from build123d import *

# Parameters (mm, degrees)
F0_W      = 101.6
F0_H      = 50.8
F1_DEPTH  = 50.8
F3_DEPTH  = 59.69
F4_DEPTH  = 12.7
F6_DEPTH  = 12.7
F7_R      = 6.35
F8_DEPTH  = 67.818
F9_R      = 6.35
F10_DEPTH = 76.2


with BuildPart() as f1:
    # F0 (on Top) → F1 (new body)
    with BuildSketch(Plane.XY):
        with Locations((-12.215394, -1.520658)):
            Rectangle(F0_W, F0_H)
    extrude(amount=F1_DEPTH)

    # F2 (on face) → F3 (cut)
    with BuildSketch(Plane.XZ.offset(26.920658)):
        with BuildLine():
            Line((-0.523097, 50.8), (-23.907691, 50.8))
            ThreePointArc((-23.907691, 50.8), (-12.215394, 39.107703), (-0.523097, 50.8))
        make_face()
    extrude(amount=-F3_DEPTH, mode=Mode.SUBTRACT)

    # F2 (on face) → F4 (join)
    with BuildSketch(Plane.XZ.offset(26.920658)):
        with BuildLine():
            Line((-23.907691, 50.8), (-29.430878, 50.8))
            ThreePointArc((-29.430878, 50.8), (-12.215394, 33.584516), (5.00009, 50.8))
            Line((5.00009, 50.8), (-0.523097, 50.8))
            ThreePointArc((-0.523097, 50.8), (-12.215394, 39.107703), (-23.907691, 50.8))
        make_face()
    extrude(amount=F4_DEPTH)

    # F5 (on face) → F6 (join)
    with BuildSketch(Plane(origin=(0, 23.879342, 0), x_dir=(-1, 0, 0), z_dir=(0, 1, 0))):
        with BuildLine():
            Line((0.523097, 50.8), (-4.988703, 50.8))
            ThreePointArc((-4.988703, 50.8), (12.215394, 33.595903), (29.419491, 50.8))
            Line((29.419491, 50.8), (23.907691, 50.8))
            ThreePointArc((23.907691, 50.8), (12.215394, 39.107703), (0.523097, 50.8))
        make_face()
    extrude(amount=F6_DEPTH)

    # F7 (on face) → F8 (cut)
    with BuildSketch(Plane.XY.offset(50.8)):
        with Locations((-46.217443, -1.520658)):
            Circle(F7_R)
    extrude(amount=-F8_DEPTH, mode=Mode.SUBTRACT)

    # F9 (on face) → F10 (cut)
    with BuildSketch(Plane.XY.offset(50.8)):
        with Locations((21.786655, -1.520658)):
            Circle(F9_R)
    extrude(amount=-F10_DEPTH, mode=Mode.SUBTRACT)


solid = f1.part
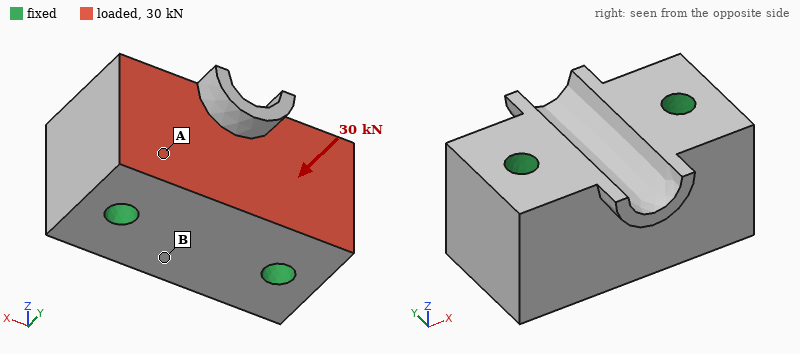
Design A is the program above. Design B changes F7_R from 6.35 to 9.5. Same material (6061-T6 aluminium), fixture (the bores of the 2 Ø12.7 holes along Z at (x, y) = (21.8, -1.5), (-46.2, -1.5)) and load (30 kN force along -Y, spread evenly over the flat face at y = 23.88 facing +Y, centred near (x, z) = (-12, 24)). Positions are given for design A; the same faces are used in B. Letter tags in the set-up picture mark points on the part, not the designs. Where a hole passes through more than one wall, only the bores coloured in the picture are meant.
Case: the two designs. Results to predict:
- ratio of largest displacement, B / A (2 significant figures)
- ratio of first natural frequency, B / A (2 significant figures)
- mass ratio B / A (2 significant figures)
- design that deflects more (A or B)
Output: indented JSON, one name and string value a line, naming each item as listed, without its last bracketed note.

{
  "ratio of largest displacement, B / A": "0.91",
  "ratio of first natural frequency, B / A": "1.1",
  "mass ratio B / A": "0.97",
  "design that deflects more": "A"
}
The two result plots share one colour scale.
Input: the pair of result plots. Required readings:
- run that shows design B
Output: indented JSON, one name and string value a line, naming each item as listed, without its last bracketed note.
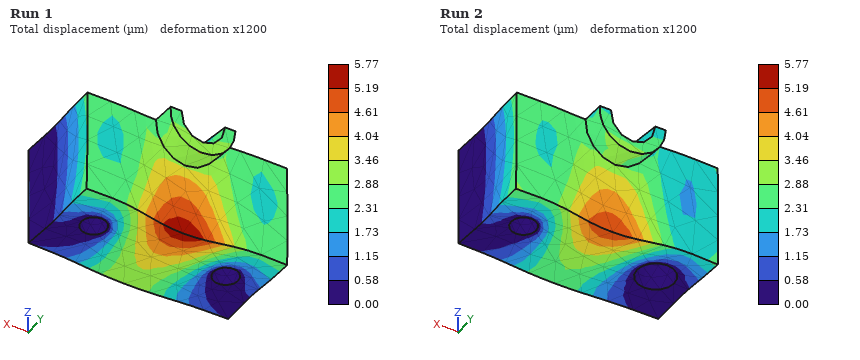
{
  "run that shows design B": "Run 2"
}
